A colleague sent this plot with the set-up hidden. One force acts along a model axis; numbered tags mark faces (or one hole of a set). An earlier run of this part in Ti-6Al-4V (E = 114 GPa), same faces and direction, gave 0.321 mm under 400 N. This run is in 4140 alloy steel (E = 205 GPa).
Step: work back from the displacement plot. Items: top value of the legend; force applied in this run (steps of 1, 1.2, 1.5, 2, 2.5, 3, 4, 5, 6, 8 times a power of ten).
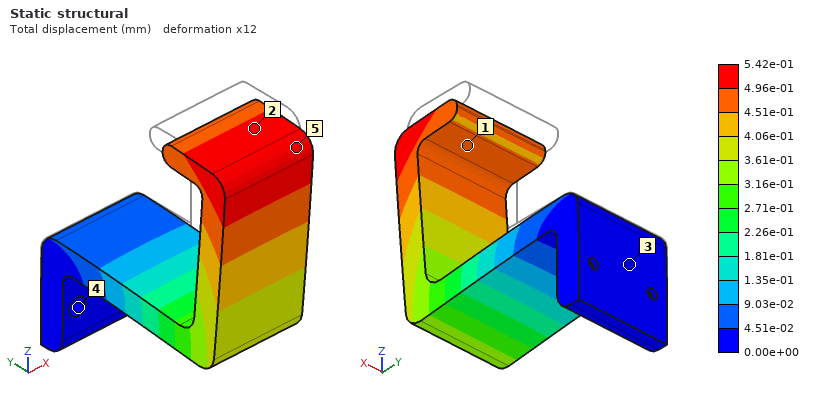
5.42e-01 mm
1.2 kN
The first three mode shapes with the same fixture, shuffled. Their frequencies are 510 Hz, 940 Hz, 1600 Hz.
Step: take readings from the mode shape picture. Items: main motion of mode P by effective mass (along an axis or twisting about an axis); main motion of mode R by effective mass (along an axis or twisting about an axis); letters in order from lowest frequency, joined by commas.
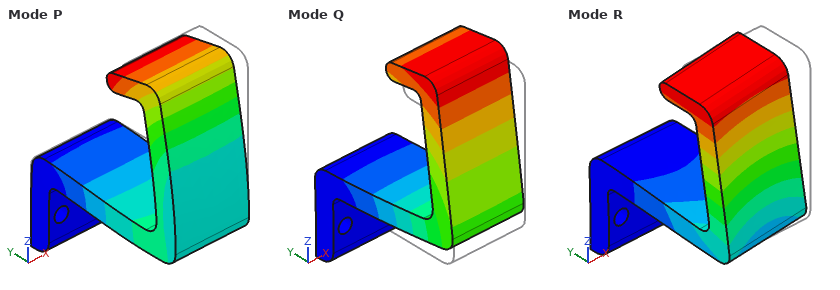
along Z
along X
Q, R, P
